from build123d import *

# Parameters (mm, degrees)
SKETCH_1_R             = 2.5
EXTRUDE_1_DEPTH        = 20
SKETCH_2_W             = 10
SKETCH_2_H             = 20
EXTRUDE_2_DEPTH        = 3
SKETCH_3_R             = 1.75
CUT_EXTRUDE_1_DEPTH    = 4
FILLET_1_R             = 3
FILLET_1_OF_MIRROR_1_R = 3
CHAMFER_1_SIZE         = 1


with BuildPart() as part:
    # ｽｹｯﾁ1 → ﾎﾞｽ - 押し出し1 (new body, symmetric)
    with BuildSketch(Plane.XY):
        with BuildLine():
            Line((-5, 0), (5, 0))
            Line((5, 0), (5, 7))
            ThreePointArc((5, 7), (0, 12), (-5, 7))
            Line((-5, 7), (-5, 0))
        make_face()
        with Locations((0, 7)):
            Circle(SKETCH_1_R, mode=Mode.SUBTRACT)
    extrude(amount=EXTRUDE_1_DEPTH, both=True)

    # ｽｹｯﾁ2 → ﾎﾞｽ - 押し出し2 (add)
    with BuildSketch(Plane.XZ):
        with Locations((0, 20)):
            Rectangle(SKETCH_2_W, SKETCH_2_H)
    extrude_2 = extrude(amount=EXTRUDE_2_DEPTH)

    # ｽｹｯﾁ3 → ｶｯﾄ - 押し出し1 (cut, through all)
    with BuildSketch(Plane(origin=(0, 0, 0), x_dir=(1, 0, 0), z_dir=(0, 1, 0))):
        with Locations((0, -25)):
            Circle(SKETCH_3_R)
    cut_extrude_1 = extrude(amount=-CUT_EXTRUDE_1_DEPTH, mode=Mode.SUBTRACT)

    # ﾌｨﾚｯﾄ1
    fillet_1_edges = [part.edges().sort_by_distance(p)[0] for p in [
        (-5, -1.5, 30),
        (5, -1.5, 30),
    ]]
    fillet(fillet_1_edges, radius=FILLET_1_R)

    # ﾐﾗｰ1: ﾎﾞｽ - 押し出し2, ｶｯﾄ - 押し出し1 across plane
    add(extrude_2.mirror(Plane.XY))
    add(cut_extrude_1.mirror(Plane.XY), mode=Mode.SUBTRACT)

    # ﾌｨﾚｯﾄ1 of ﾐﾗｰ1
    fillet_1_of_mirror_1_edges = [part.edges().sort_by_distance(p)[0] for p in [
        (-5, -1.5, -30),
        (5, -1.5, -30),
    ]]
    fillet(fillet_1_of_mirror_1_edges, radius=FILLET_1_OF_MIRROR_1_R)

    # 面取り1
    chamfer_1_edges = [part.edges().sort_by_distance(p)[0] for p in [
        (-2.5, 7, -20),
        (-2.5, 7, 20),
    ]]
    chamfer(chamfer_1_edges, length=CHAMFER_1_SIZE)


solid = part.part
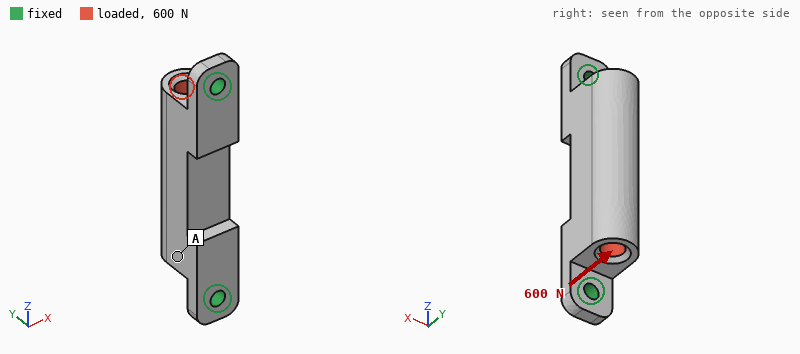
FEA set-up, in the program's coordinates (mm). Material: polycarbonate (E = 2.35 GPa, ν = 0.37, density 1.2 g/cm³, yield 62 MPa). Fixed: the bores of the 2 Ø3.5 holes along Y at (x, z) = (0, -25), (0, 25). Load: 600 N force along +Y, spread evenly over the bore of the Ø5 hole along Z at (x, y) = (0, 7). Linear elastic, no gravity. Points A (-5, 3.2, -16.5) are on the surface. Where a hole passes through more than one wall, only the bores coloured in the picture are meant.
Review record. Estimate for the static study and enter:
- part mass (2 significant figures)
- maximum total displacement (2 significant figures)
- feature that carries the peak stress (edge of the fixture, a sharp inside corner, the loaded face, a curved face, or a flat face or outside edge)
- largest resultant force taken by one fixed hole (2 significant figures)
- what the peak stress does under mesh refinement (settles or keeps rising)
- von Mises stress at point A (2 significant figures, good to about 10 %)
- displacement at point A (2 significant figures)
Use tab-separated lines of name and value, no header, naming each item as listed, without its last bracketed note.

part mass	5.6 g
maximum total displacement	0.31 mm
feature that carries the peak stress	edge of the fixture
largest resultant force taken by one fixed hole	430 N
what the peak stress does under mesh refinement	keeps rising
von Mises stress at point A	8.8 MPa
displacement at point A	0.20 mm
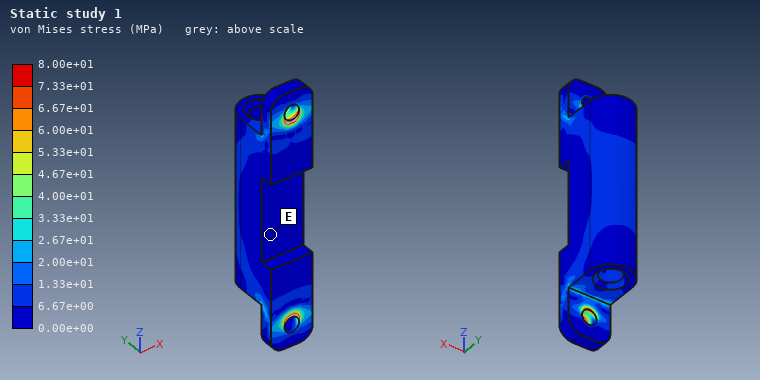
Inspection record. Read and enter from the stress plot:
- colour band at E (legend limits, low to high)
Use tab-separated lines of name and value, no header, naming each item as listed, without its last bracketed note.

colour band at E	0.00e+00 to 6.67e+00 MPa
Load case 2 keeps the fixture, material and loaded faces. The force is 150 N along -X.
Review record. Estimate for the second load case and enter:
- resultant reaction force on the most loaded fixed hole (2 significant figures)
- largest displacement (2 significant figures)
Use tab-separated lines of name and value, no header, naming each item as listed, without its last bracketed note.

resultant reaction force on the most loaded fixed hole	75 N
largest displacement	0.63 mm
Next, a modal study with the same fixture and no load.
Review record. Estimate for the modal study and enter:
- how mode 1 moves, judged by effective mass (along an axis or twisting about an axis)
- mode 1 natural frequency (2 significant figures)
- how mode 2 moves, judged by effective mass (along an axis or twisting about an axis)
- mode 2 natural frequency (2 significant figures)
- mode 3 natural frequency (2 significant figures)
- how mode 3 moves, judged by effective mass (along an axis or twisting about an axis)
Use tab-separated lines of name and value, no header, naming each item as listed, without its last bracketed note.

how mode 1 moves, judged by effective mass	along X
mode 1 natural frequency	1600 Hz
how mode 2 moves, judged by effective mass	along Y
mode 2 natural frequency	3500 Hz
mode 3 natural frequency	4800 Hz
how mode 3 moves, judged by effective mass	along X
